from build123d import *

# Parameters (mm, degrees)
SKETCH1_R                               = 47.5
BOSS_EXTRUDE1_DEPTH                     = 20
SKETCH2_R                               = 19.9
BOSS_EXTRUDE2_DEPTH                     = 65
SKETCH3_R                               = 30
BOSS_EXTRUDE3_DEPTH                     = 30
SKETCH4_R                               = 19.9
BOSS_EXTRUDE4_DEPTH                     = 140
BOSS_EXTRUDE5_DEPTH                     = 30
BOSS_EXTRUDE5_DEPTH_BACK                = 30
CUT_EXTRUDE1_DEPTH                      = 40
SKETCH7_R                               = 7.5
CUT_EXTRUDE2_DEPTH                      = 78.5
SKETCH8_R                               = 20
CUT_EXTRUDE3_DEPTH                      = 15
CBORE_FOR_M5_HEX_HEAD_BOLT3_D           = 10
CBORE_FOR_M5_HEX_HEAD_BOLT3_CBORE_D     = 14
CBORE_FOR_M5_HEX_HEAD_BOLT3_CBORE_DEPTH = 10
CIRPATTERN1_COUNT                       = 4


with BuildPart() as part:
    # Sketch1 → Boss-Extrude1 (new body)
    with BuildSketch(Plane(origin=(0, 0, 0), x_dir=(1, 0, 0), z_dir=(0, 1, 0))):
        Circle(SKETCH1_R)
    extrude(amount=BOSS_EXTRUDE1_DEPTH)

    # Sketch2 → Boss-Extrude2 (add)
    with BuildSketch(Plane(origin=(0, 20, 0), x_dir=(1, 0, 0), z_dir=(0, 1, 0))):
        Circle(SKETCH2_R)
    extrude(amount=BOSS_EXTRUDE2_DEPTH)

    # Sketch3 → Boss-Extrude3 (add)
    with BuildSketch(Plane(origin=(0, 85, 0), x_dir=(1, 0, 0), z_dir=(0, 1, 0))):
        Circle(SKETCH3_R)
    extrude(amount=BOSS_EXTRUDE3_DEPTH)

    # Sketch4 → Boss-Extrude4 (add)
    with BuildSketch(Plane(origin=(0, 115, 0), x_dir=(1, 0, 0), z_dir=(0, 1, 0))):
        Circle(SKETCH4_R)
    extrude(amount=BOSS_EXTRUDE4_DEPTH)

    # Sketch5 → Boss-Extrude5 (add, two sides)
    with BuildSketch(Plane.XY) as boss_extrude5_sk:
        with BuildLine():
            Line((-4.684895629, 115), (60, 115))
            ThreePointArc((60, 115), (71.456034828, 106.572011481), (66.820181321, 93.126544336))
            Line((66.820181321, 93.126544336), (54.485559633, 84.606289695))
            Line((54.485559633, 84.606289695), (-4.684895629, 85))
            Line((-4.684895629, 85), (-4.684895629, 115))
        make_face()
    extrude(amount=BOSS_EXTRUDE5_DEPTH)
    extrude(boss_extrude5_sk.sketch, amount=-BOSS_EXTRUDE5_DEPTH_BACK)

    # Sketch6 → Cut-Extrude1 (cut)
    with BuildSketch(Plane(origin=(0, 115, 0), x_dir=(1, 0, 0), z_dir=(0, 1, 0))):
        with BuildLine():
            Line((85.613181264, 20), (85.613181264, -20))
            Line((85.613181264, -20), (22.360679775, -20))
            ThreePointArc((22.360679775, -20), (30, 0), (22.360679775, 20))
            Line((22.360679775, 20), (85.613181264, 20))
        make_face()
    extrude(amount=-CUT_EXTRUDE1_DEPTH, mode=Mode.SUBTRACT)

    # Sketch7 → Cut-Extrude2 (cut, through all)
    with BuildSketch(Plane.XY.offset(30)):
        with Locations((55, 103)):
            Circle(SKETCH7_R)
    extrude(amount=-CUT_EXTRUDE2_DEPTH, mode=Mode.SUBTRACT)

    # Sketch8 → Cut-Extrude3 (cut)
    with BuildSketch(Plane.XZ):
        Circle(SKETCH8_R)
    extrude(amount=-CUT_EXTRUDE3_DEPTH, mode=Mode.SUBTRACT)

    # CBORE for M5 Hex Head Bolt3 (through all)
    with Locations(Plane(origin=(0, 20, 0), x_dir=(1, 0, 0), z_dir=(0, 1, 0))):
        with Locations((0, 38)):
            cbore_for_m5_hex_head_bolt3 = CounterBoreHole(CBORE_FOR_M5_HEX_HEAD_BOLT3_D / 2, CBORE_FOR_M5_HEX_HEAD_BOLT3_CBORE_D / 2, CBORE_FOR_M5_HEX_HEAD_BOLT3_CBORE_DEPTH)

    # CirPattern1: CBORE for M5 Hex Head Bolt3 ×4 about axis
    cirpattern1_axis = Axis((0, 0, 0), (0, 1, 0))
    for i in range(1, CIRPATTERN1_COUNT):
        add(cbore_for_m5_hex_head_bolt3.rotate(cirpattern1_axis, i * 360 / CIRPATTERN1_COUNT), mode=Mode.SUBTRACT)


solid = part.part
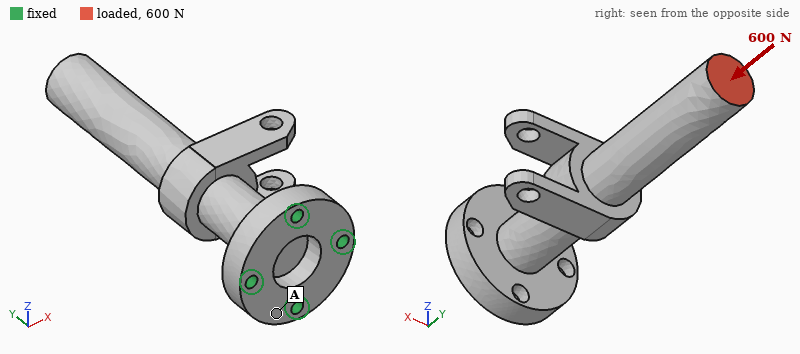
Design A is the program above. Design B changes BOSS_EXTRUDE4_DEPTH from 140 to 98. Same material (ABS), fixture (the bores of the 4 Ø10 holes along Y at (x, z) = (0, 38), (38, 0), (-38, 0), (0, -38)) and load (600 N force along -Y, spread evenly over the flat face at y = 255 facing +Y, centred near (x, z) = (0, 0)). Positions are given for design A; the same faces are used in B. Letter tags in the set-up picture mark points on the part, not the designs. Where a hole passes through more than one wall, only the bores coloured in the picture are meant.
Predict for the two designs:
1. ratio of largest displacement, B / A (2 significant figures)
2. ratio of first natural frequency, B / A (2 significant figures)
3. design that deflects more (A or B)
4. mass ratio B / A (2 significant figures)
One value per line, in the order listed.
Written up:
0.87
1.4
A
0.89
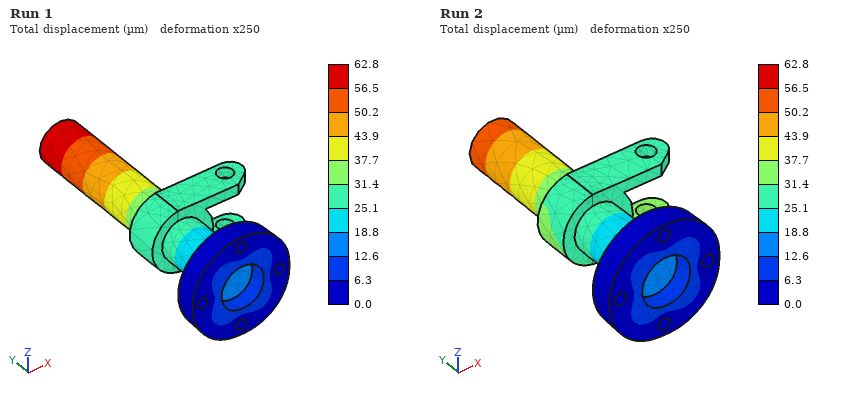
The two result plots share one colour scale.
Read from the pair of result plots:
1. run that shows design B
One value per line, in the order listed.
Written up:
Run 2
